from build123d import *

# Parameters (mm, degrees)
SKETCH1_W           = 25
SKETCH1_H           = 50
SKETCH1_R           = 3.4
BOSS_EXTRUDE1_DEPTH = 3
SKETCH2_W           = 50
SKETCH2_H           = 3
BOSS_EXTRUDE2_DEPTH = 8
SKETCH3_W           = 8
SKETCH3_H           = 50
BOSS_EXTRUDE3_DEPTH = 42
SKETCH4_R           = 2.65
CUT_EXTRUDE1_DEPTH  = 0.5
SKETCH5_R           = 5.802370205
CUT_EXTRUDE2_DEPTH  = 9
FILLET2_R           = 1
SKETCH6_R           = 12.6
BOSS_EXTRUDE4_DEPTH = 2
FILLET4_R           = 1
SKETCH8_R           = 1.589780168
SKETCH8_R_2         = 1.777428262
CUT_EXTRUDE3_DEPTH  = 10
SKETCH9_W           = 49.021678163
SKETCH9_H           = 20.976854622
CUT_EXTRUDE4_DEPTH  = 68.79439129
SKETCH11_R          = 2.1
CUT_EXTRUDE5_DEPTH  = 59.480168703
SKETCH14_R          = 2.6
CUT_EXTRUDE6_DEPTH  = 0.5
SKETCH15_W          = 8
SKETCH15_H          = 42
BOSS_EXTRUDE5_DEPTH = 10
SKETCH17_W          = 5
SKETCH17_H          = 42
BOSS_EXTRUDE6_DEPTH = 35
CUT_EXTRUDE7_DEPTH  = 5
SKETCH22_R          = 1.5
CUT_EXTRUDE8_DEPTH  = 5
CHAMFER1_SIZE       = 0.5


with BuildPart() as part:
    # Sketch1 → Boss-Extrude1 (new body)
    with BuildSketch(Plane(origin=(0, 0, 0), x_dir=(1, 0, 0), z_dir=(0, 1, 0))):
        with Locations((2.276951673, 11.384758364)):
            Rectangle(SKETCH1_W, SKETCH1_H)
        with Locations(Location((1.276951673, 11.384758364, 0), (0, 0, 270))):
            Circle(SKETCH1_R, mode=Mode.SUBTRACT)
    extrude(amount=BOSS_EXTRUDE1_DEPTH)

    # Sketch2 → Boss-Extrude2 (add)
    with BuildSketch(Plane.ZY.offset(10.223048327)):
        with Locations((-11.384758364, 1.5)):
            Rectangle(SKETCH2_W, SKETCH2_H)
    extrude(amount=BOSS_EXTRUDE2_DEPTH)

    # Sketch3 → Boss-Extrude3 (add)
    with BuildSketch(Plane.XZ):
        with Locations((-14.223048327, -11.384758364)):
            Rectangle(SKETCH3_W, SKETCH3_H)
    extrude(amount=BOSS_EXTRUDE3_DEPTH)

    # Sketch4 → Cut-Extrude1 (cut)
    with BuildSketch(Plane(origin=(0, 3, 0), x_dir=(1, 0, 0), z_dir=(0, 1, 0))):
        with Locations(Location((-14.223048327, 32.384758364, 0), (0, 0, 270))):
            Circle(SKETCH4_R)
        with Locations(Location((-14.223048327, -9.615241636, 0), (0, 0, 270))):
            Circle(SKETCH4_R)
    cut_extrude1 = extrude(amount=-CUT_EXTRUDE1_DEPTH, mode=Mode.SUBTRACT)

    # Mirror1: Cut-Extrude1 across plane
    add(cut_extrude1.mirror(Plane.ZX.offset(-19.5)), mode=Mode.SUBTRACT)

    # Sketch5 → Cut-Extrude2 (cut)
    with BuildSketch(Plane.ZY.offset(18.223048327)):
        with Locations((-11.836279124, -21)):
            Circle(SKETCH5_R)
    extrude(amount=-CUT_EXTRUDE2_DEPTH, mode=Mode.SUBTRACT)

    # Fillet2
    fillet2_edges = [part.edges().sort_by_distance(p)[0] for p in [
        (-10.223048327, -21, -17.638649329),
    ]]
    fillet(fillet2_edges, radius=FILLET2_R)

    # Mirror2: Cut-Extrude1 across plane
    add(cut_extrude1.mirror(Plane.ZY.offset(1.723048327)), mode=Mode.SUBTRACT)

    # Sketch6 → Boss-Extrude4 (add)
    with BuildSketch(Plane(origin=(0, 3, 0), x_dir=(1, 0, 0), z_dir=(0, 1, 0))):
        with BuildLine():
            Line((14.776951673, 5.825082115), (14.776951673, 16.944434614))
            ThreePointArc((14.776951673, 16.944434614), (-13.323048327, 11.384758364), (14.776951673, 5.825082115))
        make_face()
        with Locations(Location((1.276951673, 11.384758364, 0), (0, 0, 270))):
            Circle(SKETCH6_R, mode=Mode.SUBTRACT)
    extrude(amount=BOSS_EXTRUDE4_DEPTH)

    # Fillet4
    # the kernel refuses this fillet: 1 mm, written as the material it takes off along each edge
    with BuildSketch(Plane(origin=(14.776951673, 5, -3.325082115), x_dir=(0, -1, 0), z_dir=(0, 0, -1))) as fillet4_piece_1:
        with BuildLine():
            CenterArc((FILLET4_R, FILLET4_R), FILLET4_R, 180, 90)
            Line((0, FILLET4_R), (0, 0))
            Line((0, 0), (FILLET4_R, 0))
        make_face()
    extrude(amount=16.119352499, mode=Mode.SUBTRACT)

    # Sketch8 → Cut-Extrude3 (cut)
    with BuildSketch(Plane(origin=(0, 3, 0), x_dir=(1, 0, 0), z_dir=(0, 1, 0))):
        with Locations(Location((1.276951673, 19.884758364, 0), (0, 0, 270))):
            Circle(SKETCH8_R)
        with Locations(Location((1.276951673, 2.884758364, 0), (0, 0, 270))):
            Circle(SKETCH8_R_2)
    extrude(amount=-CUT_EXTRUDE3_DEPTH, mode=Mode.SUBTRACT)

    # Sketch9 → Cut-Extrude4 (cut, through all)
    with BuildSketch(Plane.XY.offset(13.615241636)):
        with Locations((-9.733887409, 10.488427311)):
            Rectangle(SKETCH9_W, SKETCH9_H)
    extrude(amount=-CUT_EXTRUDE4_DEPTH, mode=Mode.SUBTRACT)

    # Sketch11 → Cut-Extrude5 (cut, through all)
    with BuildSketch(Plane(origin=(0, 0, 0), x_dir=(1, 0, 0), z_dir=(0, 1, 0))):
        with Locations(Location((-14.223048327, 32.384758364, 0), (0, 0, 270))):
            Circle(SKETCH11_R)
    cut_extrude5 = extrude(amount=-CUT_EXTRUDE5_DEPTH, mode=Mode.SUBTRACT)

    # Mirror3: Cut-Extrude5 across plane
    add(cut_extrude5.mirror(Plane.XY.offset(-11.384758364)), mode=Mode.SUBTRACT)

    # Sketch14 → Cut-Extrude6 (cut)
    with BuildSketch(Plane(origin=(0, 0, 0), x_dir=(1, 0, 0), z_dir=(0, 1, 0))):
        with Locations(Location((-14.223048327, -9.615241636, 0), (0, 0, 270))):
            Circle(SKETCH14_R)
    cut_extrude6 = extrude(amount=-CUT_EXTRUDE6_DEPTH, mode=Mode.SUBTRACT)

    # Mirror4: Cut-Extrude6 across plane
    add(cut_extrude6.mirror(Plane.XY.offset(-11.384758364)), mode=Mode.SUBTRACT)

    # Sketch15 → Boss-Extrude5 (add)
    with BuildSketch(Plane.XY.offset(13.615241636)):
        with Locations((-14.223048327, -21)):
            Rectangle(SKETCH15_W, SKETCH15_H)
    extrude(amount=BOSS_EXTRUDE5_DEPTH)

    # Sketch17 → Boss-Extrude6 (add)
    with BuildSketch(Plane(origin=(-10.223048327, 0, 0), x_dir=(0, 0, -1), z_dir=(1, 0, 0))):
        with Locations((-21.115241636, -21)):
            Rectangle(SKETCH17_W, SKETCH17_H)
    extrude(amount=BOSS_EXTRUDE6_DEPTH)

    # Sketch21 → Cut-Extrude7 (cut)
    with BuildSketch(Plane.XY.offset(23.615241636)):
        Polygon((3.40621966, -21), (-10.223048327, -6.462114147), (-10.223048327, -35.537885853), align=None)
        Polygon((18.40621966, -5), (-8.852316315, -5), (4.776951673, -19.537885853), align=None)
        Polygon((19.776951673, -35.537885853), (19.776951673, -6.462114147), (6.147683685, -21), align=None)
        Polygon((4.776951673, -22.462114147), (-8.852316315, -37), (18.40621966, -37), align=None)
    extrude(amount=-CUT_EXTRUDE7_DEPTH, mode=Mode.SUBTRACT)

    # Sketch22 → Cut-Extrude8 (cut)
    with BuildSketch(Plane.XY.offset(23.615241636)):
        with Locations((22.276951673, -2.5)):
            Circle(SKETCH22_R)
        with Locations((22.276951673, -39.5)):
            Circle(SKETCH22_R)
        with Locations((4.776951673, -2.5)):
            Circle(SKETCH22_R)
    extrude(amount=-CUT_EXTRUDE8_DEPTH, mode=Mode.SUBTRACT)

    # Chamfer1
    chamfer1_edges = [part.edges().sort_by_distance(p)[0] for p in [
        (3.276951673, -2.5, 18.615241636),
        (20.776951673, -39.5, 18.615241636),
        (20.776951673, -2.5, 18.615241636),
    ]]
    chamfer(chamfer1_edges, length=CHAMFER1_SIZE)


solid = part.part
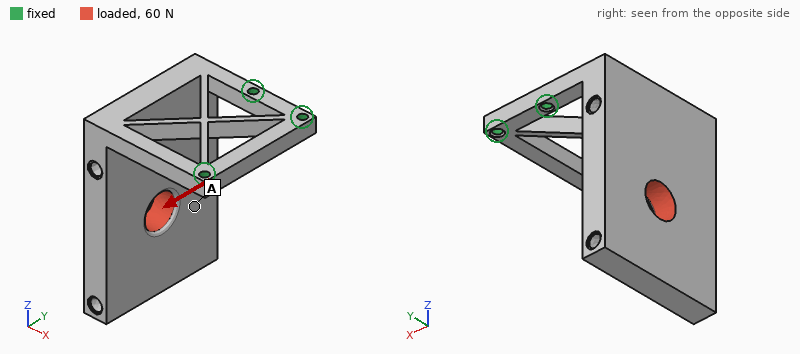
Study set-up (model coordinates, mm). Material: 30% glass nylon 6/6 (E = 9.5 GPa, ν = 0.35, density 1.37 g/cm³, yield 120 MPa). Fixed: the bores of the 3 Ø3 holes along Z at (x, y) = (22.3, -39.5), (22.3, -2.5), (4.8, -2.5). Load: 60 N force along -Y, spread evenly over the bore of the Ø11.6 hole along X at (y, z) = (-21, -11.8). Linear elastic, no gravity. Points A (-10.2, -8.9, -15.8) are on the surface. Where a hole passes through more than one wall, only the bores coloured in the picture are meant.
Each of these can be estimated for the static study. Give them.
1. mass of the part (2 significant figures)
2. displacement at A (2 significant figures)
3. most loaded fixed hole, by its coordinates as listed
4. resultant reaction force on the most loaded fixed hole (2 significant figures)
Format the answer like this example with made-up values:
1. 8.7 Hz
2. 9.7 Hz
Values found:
1. 29 g
2. 0.49 mm
3. (22.3, -39.5)
4. 69 N
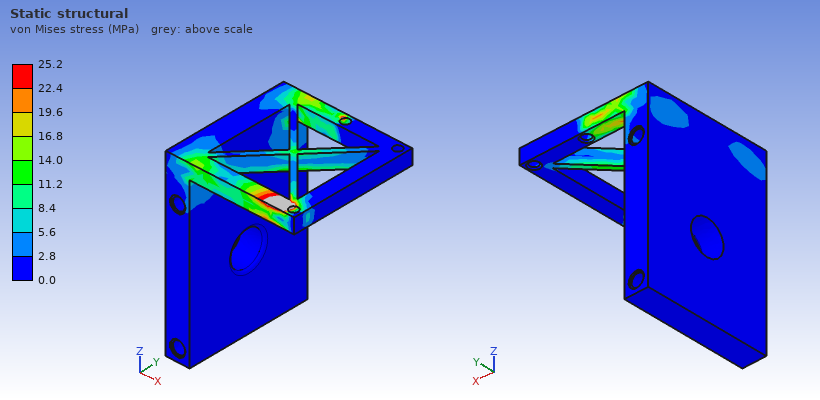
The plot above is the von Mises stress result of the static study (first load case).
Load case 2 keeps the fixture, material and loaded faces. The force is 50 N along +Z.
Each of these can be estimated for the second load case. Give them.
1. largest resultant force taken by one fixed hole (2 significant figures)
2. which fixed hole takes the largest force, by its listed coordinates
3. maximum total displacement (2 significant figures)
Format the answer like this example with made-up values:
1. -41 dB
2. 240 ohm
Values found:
1. 34 N
2. (4.8, -2.5)
3. 0.95 mm
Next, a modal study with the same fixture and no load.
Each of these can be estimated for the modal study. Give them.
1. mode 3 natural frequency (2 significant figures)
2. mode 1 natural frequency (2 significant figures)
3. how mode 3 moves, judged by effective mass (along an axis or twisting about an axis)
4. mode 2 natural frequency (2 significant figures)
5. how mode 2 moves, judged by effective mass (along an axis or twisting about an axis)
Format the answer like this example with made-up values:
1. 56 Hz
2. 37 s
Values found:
1. 1200 Hz
2. 200 Hz
3. along Z
4. 420 Hz
5. along Y
